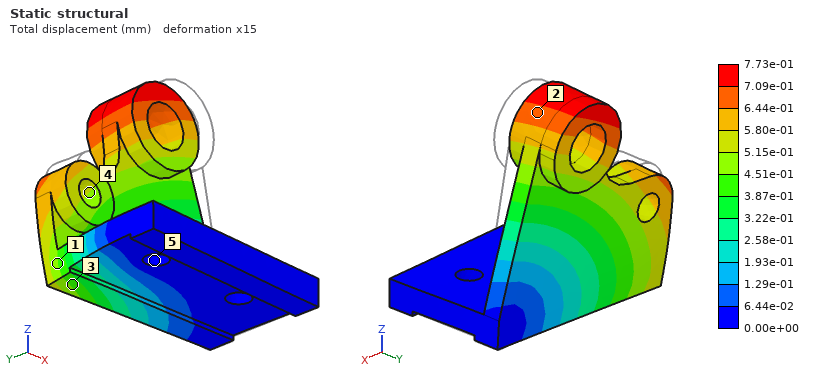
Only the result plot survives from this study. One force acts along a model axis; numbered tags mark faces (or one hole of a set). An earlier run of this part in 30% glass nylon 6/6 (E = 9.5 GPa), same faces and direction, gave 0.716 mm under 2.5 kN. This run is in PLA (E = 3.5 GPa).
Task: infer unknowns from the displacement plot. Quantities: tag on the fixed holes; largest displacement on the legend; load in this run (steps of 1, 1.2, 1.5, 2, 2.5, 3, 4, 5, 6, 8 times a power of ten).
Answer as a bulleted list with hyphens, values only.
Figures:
- 5
- 7.73e-01 mm
- 1 kN
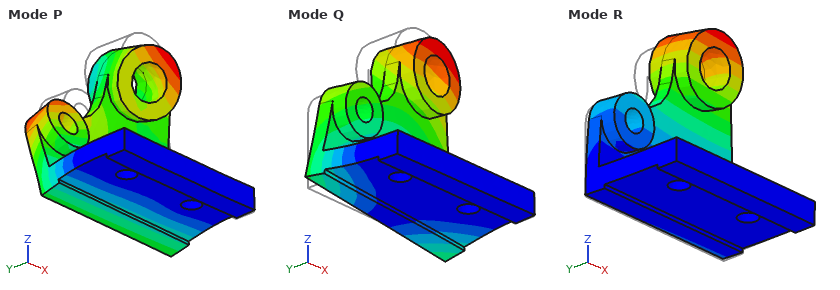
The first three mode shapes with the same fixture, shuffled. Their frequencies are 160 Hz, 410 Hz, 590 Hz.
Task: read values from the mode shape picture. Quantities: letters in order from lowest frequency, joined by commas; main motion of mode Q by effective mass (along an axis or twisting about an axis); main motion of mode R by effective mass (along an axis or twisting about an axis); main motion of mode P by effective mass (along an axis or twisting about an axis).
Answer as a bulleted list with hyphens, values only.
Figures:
- R, Q, P
- along X
- along Y
- along Z
